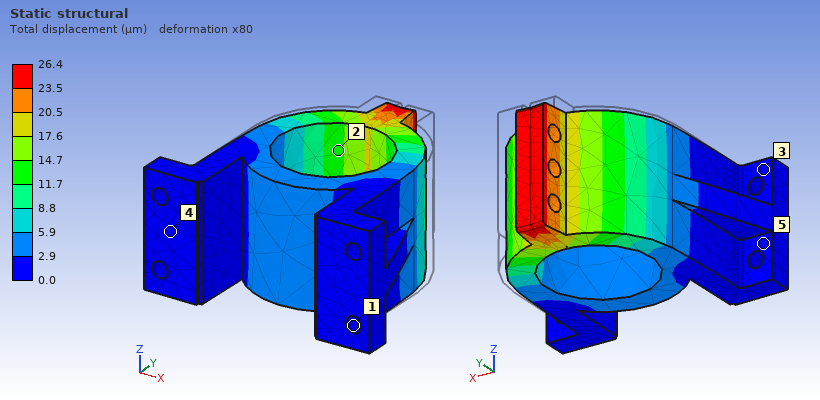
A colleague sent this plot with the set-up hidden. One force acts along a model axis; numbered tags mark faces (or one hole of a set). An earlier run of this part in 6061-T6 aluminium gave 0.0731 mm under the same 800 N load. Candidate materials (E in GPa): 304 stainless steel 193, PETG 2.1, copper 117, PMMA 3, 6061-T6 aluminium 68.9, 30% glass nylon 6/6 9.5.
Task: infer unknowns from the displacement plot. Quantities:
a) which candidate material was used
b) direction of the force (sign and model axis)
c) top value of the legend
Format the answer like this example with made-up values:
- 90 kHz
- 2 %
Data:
- 304 stainless steel
- -Y
- 26.4 µm
